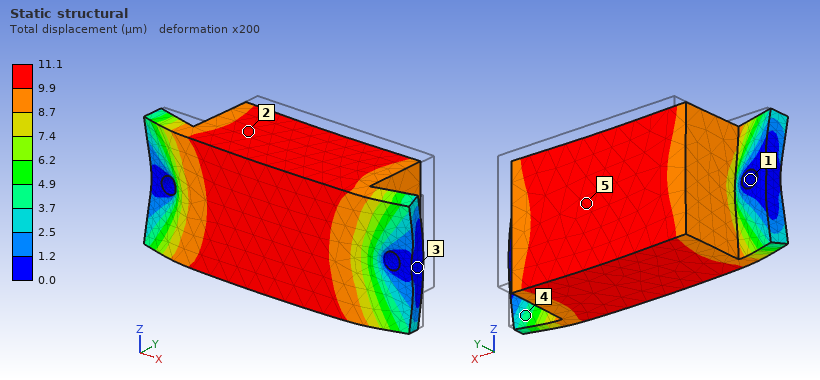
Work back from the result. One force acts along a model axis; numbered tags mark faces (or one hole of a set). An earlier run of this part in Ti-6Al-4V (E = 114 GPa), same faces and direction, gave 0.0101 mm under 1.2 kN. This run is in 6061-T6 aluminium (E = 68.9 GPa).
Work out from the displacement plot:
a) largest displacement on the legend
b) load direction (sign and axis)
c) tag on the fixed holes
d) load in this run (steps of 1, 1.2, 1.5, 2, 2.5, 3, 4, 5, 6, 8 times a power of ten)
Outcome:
11.1 µm
-Y
1
800 N
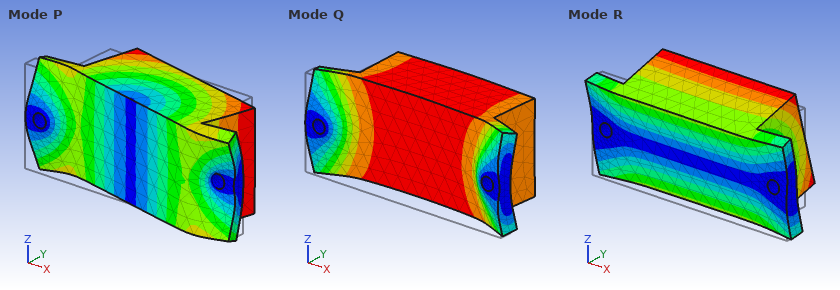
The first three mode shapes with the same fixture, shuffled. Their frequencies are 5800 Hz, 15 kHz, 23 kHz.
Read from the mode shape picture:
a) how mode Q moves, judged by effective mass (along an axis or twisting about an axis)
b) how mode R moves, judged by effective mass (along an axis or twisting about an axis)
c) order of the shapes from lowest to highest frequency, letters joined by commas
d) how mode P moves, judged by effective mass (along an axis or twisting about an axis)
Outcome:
along Y
along Z
R, Q, P
along X
